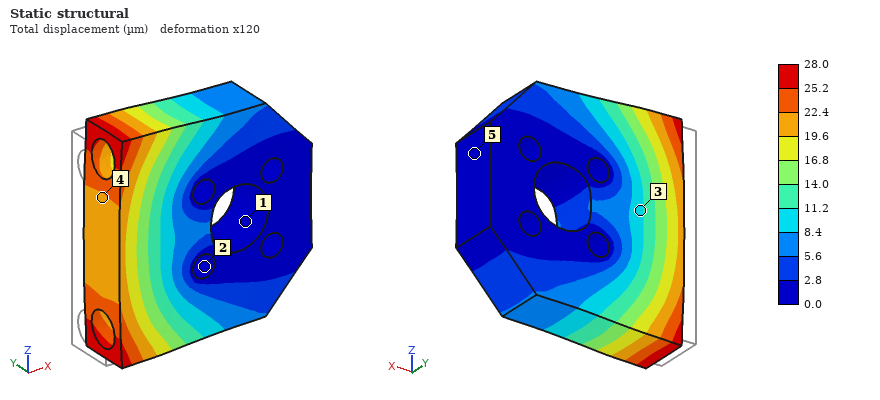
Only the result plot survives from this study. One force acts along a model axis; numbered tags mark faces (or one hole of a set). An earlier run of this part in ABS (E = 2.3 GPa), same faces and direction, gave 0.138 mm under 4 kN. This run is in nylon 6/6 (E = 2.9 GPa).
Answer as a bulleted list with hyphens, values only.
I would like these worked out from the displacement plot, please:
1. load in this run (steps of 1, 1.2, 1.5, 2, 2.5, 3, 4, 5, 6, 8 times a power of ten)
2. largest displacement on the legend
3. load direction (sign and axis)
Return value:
- 1 kN
- 28.0 µm
- +X
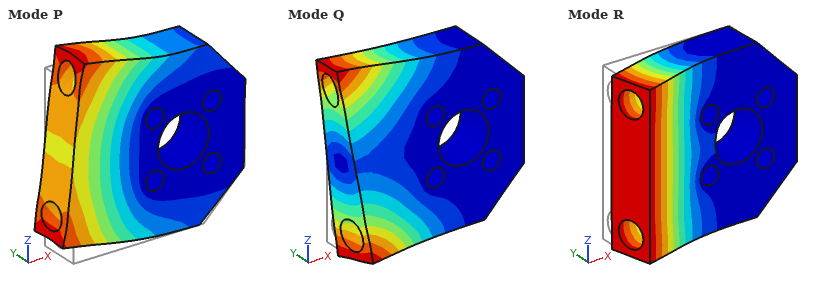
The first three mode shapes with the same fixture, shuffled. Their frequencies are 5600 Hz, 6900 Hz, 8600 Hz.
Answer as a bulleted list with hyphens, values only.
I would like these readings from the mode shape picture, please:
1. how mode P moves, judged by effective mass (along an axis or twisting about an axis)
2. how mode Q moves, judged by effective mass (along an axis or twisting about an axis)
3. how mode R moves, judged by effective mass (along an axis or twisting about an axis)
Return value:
- along Z
- twisting about X
- along Y
